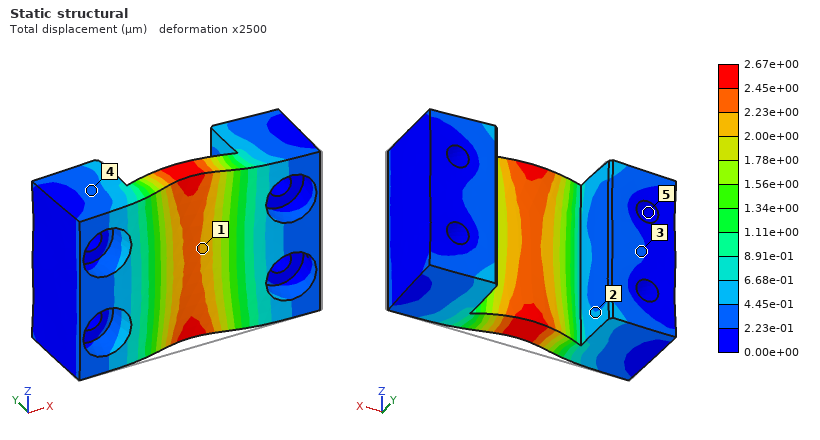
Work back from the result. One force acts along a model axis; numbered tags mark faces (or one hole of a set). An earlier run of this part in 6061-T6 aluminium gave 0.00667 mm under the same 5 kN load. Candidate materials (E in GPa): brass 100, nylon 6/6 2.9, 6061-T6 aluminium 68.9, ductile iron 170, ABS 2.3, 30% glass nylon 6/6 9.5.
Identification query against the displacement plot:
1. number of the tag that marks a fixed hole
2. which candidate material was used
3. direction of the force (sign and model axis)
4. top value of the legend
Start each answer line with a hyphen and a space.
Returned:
- 5
- ductile iron
- +Y
- 2.67e+00 µm
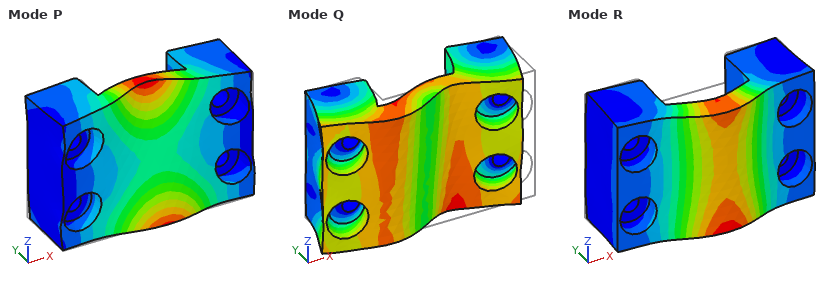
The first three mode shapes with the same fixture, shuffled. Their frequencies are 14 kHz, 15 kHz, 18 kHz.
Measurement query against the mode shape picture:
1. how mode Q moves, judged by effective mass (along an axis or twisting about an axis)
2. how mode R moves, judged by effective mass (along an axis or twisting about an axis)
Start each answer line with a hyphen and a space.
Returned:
- along X
- along Y
